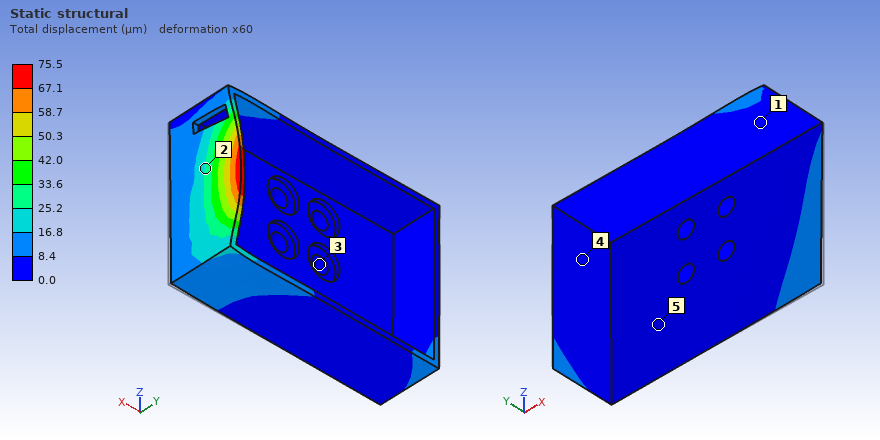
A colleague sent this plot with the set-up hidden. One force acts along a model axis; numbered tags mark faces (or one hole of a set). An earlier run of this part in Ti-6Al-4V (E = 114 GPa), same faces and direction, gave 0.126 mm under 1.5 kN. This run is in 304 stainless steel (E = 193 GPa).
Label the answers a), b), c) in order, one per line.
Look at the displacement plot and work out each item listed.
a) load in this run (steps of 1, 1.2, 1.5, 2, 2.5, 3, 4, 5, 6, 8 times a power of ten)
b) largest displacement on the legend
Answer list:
a) 1.5 kN
b) 75.5 µm
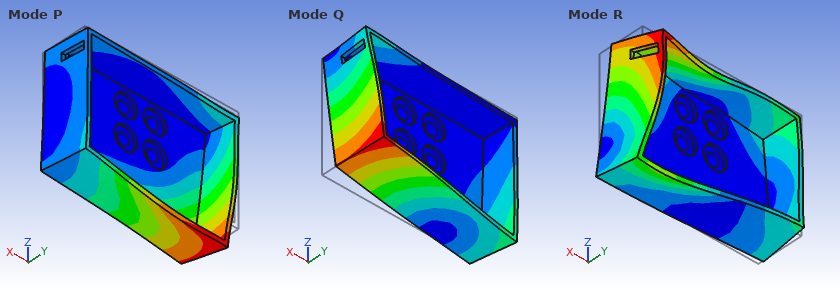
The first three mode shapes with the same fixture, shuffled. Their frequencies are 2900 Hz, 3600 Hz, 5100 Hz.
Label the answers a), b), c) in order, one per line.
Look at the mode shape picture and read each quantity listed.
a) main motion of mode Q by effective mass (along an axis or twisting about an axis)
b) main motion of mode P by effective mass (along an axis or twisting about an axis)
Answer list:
a) along Y
b) along Y
